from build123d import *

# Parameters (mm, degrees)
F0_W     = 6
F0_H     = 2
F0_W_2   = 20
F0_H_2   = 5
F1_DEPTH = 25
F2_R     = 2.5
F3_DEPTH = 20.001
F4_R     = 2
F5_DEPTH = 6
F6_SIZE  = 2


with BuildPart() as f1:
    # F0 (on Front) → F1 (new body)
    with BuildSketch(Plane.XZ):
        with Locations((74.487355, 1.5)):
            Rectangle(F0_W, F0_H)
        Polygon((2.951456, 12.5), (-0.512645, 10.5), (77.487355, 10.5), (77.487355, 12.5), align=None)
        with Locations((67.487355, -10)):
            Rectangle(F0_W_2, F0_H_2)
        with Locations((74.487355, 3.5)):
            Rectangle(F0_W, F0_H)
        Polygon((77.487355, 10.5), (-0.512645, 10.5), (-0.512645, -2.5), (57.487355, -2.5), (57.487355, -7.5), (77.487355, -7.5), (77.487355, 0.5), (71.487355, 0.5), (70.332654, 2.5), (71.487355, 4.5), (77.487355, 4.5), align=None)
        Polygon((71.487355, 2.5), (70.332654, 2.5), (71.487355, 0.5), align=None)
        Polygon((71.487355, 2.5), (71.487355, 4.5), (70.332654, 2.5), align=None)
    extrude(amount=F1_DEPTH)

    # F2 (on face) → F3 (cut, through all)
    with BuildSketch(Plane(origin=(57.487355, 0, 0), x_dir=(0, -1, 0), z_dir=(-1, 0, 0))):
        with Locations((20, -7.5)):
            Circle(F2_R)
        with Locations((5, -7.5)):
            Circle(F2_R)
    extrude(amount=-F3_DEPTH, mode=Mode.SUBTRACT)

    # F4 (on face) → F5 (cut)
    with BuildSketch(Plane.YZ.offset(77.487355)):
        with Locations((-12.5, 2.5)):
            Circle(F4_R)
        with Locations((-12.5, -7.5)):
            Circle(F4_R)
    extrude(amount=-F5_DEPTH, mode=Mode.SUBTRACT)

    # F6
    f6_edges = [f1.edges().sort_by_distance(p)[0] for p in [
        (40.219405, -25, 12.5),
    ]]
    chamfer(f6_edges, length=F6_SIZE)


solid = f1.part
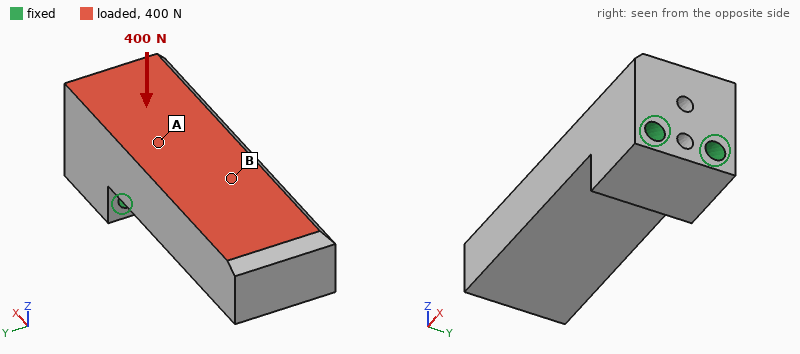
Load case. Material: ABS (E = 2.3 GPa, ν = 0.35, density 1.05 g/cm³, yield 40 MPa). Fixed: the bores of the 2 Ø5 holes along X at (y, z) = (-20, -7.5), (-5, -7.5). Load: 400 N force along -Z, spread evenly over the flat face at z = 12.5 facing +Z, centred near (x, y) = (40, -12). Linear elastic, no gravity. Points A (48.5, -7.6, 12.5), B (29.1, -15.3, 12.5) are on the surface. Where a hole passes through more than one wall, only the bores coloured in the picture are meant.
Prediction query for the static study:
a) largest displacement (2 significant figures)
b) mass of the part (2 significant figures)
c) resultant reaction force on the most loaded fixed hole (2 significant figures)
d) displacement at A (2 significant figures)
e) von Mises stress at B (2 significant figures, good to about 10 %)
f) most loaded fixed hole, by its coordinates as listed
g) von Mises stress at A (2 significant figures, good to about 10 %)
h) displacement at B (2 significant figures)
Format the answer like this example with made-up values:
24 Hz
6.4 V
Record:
0.82 mm
35 g
240 N
0.16 mm
2.1 MPa
(-5, -7.5)
6.2 MPa
0.39 mm
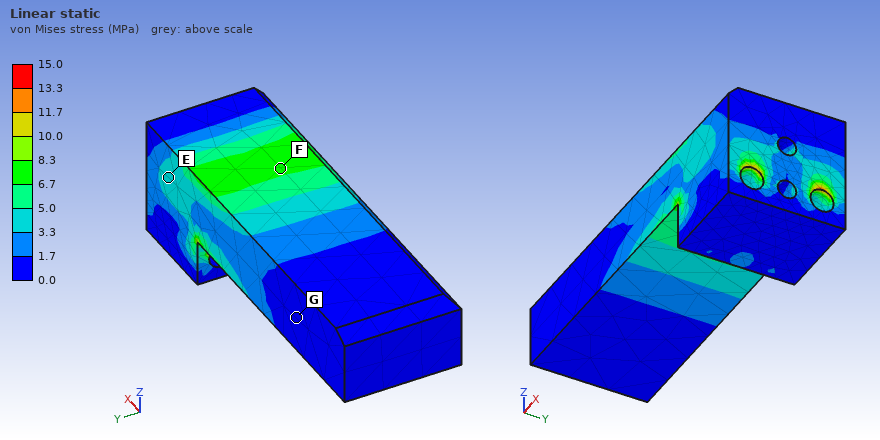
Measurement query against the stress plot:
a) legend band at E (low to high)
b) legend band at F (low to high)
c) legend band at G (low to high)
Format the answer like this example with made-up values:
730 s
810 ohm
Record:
3.3 to 5.0 MPa
6.7 to 8.3 MPa
0.0 to 1.7 MPa
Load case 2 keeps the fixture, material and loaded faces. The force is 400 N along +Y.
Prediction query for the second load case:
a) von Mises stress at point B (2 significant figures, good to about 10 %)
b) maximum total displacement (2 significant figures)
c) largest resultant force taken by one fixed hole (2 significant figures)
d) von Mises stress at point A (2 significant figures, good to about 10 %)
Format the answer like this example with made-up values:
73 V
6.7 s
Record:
2.4 MPa
0.44 mm
640 N
3.2 MPa
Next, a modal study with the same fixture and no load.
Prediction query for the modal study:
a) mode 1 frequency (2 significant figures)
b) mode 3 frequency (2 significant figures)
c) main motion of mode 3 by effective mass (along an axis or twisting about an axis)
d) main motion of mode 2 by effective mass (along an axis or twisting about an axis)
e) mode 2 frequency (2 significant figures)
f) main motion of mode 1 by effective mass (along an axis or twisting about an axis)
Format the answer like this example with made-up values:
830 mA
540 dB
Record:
750 Hz
2900 Hz
twisting about X
along Y
1000 Hz
along Z
